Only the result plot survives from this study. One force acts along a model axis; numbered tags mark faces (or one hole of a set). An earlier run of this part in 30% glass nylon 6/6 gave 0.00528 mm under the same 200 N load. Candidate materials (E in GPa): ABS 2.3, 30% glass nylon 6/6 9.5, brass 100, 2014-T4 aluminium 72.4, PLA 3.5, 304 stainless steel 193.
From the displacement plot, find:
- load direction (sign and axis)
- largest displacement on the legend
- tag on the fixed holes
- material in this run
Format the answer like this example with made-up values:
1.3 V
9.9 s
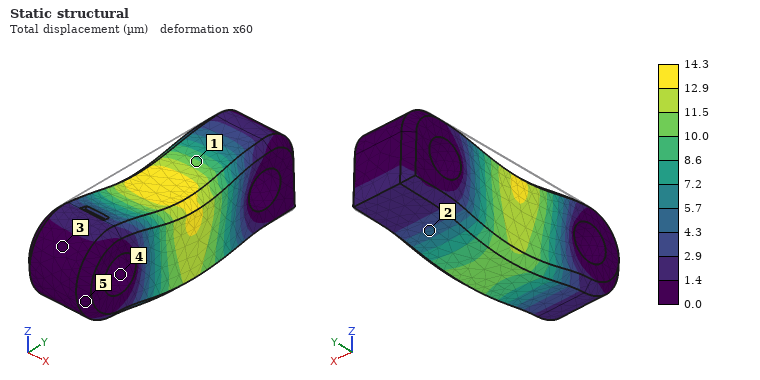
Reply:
-Z
14.3 µm
4
PLA
